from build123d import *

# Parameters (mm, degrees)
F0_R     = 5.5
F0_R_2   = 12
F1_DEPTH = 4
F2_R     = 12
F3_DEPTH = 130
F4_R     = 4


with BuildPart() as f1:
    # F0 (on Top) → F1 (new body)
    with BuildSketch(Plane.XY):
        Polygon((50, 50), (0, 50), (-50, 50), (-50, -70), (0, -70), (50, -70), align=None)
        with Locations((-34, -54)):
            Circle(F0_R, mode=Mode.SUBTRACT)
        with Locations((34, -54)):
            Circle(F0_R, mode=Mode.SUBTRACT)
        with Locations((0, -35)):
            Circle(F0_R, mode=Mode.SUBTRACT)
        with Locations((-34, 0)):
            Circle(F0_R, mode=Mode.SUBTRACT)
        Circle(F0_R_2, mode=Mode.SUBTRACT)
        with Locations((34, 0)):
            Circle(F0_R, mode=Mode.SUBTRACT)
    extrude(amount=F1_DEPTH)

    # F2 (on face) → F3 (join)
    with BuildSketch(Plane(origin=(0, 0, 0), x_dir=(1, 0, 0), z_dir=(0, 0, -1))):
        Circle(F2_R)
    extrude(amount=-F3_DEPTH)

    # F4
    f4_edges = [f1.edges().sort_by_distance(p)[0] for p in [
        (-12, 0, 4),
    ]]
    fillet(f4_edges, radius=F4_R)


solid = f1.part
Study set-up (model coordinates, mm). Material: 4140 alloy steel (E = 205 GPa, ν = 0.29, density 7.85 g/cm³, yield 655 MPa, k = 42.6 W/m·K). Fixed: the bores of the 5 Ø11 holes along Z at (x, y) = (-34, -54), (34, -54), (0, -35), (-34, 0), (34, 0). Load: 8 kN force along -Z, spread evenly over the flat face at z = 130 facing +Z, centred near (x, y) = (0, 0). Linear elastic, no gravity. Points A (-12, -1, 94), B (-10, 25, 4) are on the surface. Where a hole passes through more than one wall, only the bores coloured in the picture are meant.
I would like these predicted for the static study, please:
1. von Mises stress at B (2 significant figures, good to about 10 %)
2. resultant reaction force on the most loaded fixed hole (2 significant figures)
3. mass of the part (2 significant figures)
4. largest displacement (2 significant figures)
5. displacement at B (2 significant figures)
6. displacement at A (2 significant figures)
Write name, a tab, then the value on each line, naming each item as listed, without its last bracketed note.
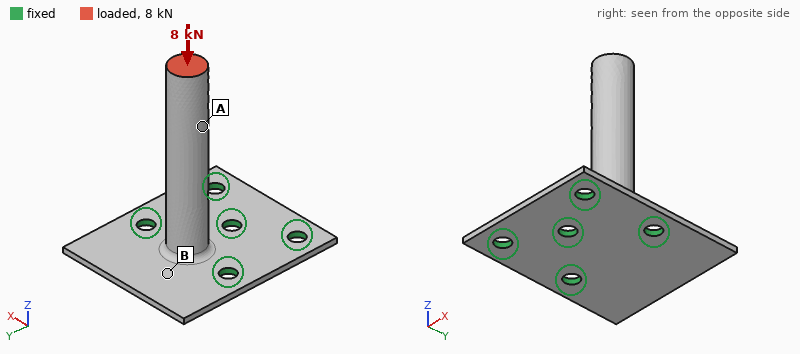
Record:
von Mises stress at B	64 MPa
resultant reaction force on the most loaded fixed hole	3.7 kN
mass of the part	810 g
largest displacement	0.26 mm
displacement at B	0.098 mm
displacement at A	0.19 mm
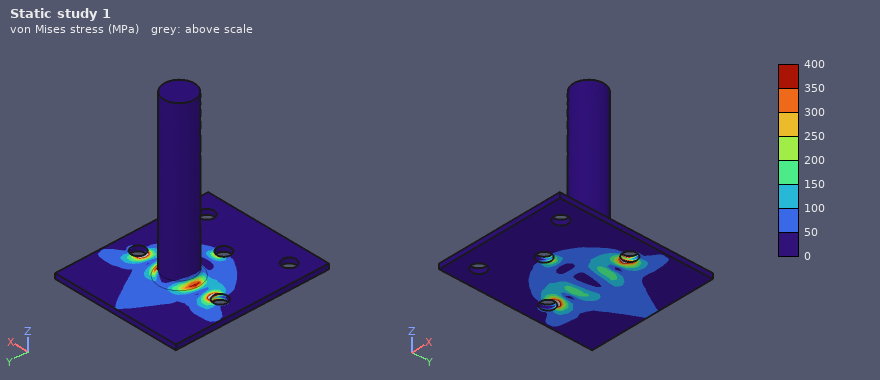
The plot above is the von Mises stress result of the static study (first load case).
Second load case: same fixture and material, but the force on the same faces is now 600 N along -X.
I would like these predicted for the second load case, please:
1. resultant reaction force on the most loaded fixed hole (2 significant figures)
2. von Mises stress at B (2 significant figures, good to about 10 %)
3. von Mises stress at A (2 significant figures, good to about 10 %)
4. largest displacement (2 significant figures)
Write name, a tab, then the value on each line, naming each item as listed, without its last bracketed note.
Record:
resultant reaction force on the most loaded fixed hole	1.6 kN
von Mises stress at B	27 MPa
von Mises stress at A	16 MPa
largest displacement	0.32 mm
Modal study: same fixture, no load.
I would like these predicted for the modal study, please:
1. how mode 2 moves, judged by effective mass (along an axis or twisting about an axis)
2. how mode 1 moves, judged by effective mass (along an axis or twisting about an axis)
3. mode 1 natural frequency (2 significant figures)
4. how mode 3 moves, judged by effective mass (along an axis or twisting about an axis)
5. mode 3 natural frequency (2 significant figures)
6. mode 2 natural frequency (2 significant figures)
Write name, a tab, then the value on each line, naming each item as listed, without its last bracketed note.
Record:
how mode 2 moves, judged by effective mass	along X
how mode 1 moves, judged by effective mass	along Y
mode 1 natural frequency	450 Hz
how mode 3 moves, judged by effective mass	along Z
mode 3 natural frequency	1700 Hz
mode 2 natural frequency	590 Hz
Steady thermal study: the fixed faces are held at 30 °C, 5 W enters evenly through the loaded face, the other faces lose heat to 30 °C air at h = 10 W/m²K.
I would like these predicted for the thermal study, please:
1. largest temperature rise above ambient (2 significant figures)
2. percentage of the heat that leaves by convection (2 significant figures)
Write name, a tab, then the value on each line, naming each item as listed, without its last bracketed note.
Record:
largest temperature rise above ambient	31 K
percentage of the heat that leaves by convection	37 %
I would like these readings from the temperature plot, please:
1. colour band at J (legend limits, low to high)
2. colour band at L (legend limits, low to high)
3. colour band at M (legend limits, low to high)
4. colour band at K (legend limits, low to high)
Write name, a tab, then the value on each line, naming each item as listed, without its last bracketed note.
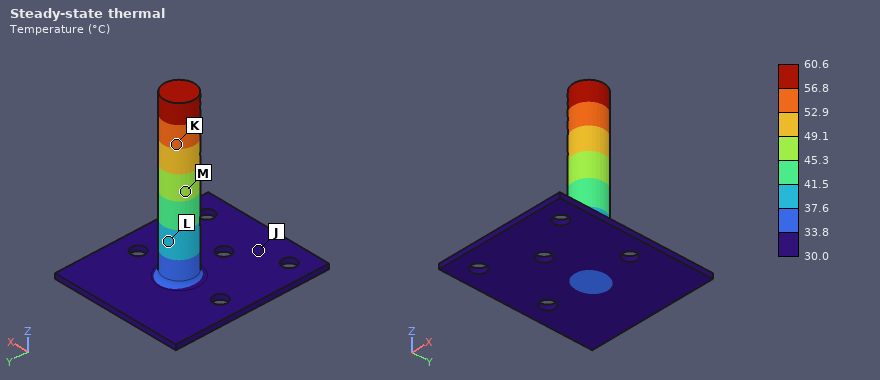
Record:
colour band at J	30.0 to 33.8 °C
colour band at L	37.6 to 41.5 °C
colour band at M	45.3 to 49.1 °C
colour band at K	52.9 to 56.8 °C
